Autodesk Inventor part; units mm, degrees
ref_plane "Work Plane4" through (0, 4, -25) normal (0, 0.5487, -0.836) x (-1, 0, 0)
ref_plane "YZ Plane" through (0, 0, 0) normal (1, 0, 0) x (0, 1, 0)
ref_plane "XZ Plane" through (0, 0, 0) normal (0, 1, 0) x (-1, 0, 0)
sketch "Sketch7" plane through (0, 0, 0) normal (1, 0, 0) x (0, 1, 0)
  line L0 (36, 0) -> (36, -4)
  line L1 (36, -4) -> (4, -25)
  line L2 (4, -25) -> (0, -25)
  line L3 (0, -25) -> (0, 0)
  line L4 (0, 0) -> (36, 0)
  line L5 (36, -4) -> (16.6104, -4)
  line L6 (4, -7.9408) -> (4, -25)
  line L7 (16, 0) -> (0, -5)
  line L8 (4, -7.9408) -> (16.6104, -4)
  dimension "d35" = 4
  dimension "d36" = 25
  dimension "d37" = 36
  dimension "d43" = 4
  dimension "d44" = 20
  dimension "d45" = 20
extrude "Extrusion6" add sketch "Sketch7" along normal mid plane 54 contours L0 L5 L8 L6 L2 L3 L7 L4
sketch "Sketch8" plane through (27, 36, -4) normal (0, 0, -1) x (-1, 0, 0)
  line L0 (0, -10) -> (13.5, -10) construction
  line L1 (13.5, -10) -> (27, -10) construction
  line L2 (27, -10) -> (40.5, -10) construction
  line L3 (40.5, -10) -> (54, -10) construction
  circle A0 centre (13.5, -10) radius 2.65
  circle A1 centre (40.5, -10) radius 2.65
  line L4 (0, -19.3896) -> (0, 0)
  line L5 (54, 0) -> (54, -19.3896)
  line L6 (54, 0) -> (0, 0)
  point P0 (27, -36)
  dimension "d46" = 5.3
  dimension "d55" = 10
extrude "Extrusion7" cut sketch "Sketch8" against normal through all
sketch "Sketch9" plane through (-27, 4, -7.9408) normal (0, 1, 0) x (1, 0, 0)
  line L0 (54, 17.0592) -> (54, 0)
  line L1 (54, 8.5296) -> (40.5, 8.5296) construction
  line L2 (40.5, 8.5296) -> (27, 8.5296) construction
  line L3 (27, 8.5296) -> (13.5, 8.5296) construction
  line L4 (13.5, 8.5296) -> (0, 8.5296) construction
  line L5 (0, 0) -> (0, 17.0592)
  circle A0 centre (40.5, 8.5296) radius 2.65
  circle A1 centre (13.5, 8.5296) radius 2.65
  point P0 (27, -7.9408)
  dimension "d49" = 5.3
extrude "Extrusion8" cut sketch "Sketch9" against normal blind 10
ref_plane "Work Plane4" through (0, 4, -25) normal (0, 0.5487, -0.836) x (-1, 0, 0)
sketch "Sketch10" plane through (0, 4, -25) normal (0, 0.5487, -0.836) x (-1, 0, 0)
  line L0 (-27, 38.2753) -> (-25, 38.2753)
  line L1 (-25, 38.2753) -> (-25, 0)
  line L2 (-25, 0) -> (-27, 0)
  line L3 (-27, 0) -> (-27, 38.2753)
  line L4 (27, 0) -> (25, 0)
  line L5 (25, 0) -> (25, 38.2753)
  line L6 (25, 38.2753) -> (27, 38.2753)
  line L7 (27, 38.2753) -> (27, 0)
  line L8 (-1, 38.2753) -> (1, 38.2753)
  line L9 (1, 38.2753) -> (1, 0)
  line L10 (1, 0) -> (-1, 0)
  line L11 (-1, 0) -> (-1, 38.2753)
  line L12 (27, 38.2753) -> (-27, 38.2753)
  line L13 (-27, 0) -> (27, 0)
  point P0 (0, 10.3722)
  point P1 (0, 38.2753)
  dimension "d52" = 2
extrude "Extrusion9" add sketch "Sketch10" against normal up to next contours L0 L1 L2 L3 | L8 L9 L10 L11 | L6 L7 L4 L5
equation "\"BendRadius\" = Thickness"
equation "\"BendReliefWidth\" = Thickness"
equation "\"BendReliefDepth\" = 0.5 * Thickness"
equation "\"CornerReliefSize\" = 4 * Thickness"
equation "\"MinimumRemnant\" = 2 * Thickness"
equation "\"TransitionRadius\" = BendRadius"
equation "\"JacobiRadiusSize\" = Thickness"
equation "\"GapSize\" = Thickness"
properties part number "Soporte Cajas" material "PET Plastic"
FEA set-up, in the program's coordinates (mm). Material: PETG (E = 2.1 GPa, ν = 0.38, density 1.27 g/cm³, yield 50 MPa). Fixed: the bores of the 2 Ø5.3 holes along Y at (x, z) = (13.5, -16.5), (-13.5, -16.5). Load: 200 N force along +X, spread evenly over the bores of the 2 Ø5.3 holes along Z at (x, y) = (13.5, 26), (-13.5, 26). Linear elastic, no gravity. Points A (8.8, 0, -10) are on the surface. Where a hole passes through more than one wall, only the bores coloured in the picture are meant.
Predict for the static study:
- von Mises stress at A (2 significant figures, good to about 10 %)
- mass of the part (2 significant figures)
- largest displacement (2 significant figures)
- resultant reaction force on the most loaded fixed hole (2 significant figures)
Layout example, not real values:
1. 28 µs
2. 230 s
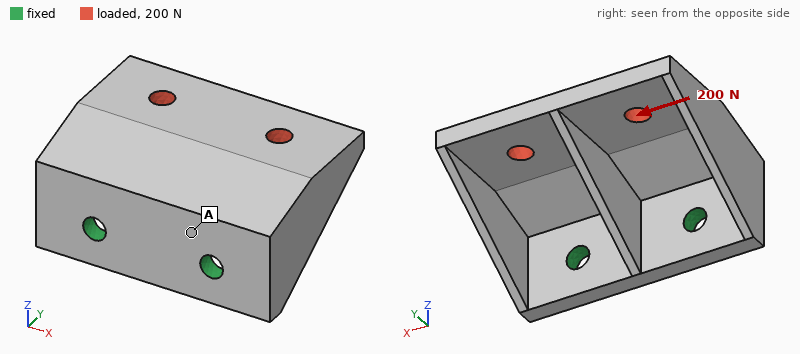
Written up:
1. 4.2 MPa
2. 17 g
3. 0.70 mm
4. 200 N
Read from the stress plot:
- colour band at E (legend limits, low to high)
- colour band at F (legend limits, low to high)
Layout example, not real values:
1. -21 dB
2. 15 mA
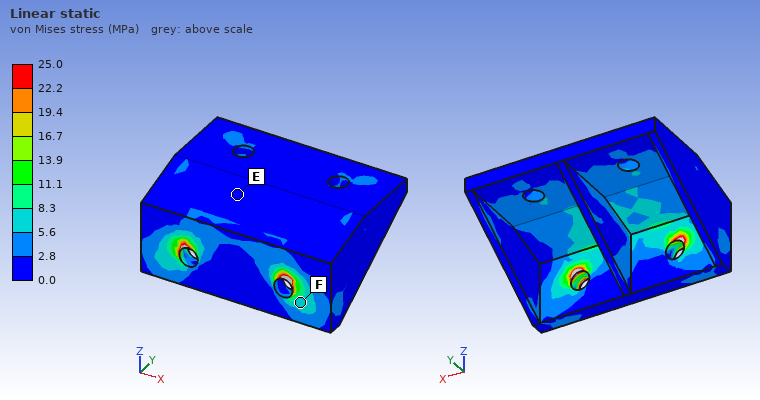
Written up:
1. 0.0 to 2.8 MPa
2. 5.6 to 8.3 MPa
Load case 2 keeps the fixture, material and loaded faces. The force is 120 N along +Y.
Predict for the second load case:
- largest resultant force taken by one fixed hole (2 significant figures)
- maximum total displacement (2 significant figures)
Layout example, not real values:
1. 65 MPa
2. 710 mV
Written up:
1. 60 N
2. 0.37 mm
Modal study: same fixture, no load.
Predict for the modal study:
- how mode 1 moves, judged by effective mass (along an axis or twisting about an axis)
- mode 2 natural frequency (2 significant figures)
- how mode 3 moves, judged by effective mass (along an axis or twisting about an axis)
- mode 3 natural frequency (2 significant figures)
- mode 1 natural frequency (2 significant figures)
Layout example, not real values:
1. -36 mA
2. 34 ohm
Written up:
1. along Z
2. 960 Hz
3. along X
4. 2000 Hz
5. 800 Hz
